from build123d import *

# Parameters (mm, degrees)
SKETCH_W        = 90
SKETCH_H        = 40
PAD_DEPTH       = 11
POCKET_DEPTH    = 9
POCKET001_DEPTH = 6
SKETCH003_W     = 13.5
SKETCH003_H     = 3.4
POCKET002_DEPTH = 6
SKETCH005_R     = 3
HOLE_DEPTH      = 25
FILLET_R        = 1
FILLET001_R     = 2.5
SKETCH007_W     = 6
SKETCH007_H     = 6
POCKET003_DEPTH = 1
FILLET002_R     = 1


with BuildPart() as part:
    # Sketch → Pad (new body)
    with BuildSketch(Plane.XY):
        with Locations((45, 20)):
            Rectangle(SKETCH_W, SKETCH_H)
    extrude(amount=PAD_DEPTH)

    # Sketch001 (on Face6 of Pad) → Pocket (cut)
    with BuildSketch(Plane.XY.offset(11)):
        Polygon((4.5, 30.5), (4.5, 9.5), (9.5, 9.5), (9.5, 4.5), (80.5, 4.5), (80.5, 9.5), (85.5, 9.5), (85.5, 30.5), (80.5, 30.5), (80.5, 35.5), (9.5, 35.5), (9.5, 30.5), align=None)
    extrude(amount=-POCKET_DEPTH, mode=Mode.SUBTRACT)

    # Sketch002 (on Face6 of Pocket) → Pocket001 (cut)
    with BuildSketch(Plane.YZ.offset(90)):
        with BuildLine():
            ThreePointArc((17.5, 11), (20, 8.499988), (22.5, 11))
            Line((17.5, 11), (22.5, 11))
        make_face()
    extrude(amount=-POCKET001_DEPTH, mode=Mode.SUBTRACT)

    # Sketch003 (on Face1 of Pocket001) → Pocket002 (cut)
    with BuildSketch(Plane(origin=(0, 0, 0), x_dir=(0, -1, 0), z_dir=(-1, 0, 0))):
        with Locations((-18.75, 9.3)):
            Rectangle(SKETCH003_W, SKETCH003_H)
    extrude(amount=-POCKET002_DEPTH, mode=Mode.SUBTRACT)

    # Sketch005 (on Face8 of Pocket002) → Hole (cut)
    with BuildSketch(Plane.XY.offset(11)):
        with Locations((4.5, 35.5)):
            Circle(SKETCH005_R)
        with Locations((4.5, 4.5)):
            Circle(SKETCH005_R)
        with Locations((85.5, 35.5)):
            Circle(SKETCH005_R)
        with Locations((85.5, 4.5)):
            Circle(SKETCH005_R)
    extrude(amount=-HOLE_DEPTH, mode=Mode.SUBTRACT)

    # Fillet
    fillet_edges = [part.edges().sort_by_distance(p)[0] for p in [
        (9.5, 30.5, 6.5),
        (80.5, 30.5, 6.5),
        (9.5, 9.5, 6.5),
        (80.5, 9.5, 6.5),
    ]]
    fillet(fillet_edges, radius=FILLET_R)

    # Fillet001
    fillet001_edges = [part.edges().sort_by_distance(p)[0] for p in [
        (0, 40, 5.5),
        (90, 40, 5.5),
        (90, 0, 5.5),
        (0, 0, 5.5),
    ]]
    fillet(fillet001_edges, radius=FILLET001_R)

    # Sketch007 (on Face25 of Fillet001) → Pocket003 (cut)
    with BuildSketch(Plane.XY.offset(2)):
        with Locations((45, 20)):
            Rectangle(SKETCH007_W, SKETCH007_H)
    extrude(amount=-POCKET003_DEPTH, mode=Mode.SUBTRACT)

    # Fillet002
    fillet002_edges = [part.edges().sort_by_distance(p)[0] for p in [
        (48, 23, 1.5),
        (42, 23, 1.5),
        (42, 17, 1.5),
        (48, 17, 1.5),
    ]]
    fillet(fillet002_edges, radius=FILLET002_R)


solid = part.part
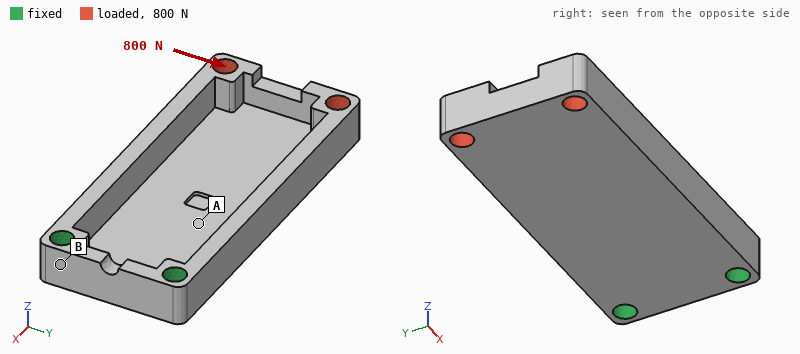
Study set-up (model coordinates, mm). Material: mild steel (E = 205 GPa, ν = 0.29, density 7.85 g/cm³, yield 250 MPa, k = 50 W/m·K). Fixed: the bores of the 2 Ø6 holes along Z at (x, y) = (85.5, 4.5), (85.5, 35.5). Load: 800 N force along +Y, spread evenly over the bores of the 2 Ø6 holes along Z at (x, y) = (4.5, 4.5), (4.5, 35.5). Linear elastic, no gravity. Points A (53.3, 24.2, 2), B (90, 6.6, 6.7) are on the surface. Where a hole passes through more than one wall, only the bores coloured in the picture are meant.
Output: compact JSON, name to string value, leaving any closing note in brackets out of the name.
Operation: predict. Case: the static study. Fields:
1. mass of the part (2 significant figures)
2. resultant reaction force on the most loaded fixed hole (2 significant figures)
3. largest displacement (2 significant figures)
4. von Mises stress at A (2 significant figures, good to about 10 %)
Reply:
{"mass of the part": "130 g", "resultant reaction force on the most loaded fixed hole": "1.9 kN", "largest displacement": "0.12 mm", "von Mises stress at A": "39 MPa"}
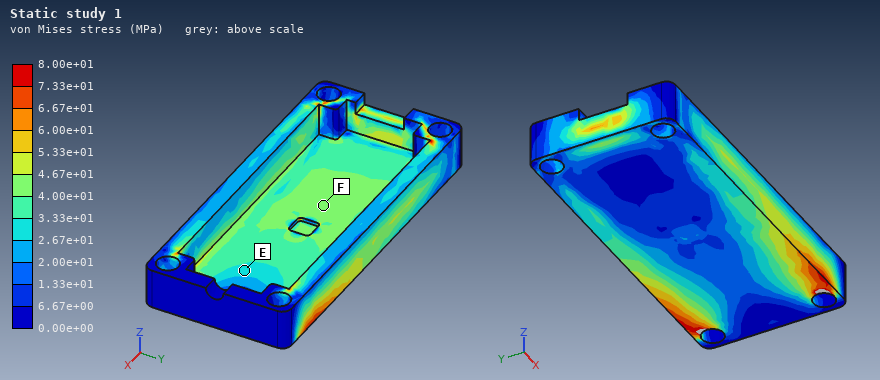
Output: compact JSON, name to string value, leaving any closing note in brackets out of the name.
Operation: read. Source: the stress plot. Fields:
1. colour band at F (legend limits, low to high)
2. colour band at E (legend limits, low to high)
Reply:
{"colour band at F": "4.00e+01 to 4.67e+01 MPa", "colour band at E": "2.67e+01 to 3.33e+01 MPa"}
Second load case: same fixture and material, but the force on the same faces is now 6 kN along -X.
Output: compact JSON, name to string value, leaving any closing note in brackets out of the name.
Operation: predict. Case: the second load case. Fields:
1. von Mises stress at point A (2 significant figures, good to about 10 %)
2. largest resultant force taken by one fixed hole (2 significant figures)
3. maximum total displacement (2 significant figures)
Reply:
{"von Mises stress at point A": "23 MPa", "largest resultant force taken by one fixed hole": "3.0 kN", "maximum total displacement": "0.10 mm"}
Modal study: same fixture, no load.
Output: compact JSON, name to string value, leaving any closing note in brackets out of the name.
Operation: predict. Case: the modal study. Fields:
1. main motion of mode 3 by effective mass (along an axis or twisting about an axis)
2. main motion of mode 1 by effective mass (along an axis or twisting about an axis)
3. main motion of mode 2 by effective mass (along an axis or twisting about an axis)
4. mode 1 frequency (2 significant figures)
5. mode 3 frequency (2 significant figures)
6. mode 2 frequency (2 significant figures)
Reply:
{"main motion of mode 3 by effective mass": "along Y", "main motion of mode 1 by effective mass": "along Z", "main motion of mode 2 by effective mass": "along Y", "mode 1 frequency": "1200 Hz", "mode 3 frequency": "4500 Hz", "mode 2 frequency": "1900 Hz"}
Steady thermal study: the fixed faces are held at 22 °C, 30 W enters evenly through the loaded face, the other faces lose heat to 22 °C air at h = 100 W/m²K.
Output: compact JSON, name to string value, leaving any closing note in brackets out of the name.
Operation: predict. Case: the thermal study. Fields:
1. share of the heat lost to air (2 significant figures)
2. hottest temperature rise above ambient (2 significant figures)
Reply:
{"share of the heat lost to air": "93 %", "hottest temperature rise above ambient": "82 K"}
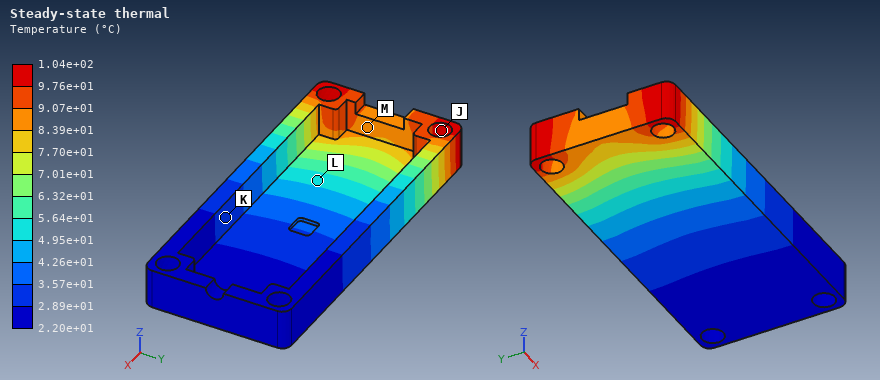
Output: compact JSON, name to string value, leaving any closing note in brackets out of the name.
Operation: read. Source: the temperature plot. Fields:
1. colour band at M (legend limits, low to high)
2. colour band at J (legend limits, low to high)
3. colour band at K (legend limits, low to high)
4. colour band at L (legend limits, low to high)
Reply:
{"colour band at M": "8.39e+01 to 9.07e+01 °C", "colour band at J": "9.76e+01 to 1.04e+02 °C", "colour band at K": "2.89e+01 to 3.57e+01 °C", "colour band at L": "4.95e+01 to 5.64e+01 °C"}
